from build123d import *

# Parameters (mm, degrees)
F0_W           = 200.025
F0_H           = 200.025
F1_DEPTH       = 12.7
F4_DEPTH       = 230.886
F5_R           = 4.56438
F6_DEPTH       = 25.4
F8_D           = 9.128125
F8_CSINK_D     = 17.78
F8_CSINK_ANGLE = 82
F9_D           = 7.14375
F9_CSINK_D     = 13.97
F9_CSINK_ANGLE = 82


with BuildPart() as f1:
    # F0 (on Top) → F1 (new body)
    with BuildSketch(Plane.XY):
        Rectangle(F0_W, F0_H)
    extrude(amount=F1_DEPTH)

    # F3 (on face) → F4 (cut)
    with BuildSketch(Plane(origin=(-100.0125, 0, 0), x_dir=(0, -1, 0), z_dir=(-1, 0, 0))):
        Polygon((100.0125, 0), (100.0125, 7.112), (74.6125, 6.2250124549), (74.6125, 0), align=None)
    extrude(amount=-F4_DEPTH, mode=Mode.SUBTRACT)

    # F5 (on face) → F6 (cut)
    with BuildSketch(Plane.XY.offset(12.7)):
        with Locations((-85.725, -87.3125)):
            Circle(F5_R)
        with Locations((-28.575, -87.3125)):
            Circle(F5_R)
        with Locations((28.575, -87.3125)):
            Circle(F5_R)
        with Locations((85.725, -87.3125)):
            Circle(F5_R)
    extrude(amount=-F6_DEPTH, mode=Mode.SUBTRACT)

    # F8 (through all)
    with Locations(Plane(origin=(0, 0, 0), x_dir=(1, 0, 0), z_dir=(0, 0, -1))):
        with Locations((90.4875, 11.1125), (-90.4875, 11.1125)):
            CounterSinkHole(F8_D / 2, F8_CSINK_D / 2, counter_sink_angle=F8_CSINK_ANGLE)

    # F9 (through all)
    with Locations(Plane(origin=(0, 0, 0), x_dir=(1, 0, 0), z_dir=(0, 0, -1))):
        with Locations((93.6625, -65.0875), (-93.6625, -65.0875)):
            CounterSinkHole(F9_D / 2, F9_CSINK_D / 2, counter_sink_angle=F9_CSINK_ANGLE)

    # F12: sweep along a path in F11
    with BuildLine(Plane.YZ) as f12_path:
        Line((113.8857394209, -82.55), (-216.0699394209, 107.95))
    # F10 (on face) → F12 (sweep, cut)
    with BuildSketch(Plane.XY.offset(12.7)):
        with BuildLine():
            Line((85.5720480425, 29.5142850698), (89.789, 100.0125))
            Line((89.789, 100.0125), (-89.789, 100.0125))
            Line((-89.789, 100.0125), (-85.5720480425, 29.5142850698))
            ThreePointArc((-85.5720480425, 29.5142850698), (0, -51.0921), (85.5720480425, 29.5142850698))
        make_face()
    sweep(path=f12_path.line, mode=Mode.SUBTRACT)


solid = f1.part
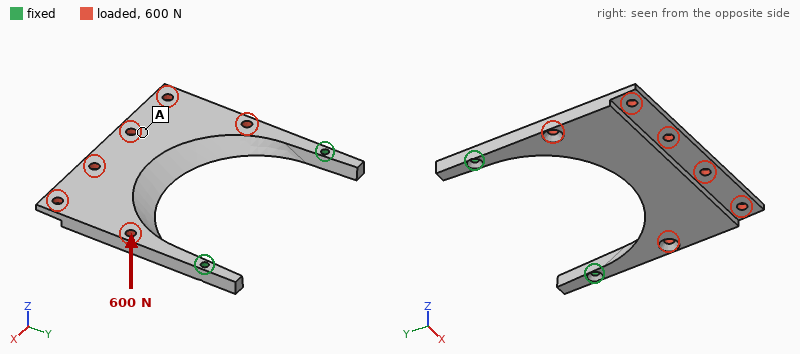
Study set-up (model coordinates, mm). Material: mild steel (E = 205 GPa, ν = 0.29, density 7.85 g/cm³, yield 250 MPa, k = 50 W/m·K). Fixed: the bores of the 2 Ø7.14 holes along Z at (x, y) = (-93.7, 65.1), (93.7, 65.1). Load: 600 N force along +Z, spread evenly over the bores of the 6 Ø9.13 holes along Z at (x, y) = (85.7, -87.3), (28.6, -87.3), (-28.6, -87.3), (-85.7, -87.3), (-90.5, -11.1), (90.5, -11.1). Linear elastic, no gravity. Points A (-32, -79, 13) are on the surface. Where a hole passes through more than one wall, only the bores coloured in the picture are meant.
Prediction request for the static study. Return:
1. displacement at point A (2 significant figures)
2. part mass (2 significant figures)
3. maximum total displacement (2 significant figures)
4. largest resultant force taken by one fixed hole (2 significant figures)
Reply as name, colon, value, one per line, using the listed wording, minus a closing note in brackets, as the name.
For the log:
displacement at point A: 0.47 mm
part mass: 1.6 kg
maximum total displacement: 0.56 mm
largest resultant force taken by one fixed hole: 300 N
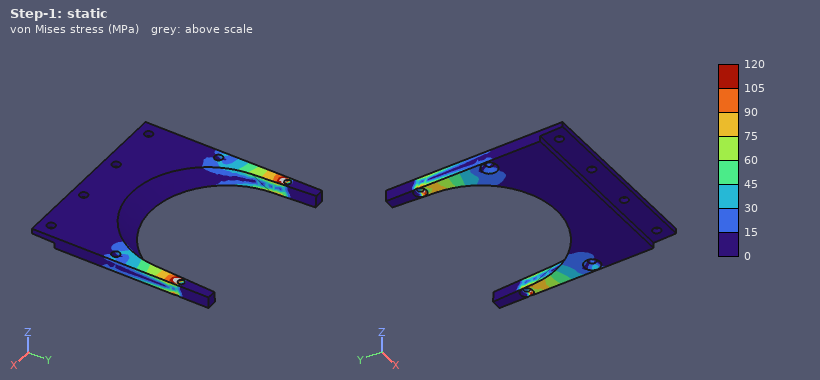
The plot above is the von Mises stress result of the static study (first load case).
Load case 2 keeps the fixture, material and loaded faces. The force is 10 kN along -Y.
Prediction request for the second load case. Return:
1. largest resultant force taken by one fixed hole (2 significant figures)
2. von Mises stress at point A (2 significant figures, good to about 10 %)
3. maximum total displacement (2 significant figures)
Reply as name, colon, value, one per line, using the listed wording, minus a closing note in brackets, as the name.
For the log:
largest resultant force taken by one fixed hole: 5.0 kN
von Mises stress at point A: 9.9 MPa
maximum total displacement: 0.31 mm
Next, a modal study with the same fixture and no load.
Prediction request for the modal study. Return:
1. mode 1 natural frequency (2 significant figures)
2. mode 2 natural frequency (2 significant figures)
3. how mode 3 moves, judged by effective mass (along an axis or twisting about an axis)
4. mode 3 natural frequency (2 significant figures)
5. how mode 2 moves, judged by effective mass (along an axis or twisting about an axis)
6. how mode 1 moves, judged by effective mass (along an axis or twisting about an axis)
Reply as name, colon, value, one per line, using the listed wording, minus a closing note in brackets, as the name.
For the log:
mode 1 natural frequency: 180 Hz
mode 2 natural frequency: 540 Hz
how mode 3 moves, judged by effective mass: along X
mode 3 natural frequency: 1000 Hz
how mode 2 moves, judged by effective mass: twisting about Y
how mode 1 moves, judged by effective mass: along Z
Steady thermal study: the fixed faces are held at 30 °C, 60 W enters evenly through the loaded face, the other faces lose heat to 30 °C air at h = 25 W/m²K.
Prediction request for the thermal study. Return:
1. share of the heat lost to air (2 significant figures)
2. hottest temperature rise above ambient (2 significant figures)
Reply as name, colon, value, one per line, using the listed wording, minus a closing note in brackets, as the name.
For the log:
share of the heat lost to air: 81 %
hottest temperature rise above ambient: 60 K
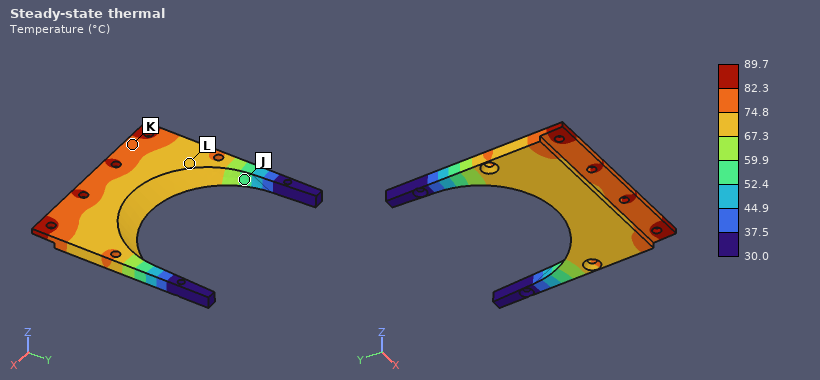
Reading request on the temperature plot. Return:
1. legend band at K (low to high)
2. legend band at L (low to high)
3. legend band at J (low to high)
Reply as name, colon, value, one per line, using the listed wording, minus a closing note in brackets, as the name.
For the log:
legend band at K: 74.8 to 82.3 °C
legend band at L: 67.3 to 74.8 °C
legend band at J: 52.4 to 59.9 °C
